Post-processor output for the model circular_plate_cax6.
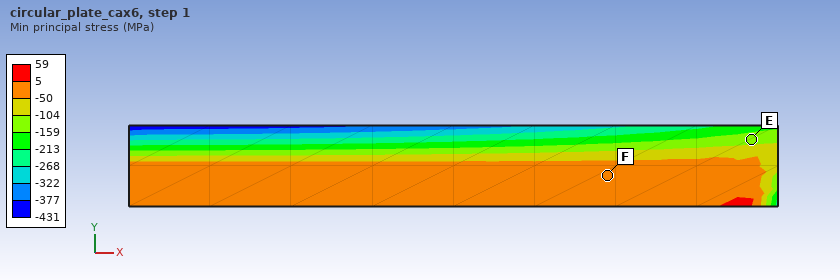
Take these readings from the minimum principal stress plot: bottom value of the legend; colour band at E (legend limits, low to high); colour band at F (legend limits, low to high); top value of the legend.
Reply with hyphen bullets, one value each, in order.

- -431 MPa
- -159 to -104 MPa
- -50 to 5 MPa
- 59 MPa
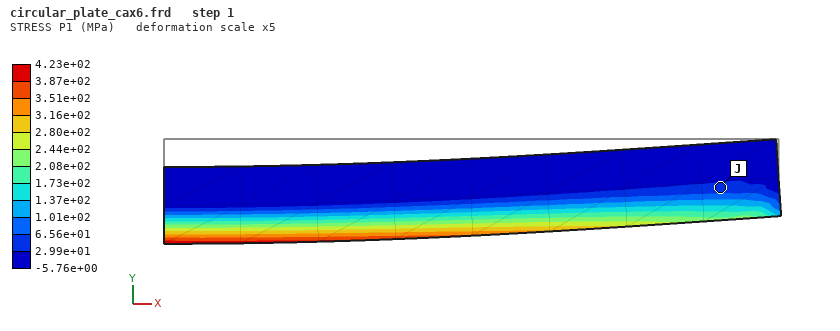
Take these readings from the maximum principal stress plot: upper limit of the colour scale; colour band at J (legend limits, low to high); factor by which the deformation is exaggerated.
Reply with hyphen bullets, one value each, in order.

- 4.23e+02 MPa
- 2.99e+01 to 6.56e+01 MPa
- 5
